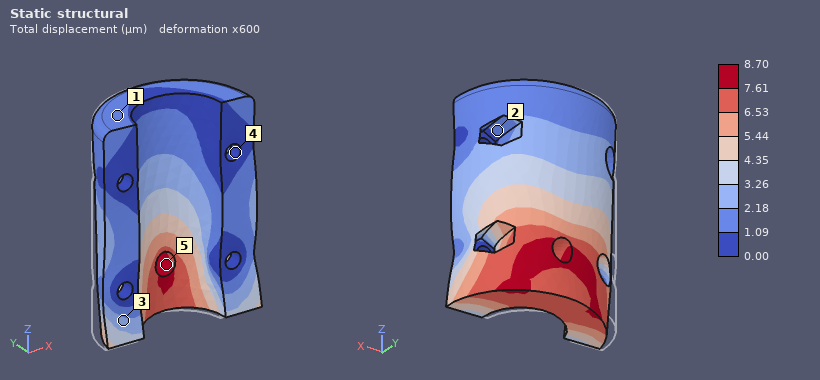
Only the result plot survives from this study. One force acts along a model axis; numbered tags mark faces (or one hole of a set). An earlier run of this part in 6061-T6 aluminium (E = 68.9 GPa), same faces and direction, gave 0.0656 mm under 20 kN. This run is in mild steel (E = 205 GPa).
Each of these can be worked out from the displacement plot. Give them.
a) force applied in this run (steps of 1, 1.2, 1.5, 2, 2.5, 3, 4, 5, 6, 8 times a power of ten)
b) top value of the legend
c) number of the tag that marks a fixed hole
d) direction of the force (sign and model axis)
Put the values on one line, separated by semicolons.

8 kN; 8.70 µm; 4; +X
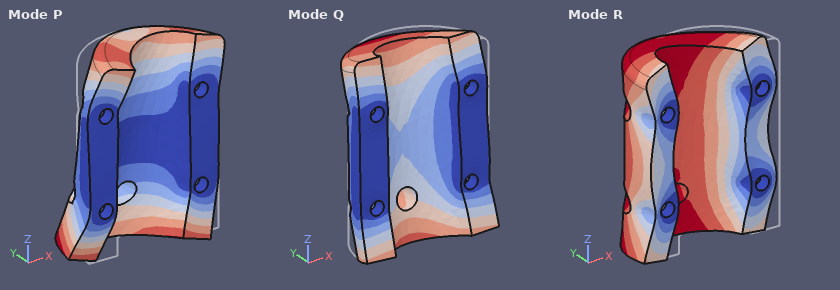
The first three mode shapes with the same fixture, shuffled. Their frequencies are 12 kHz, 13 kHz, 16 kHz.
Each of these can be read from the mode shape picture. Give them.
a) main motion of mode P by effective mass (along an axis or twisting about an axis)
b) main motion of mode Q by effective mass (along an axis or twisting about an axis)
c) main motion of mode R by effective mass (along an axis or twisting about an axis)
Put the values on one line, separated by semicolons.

twisting about Y; along Z; along X
